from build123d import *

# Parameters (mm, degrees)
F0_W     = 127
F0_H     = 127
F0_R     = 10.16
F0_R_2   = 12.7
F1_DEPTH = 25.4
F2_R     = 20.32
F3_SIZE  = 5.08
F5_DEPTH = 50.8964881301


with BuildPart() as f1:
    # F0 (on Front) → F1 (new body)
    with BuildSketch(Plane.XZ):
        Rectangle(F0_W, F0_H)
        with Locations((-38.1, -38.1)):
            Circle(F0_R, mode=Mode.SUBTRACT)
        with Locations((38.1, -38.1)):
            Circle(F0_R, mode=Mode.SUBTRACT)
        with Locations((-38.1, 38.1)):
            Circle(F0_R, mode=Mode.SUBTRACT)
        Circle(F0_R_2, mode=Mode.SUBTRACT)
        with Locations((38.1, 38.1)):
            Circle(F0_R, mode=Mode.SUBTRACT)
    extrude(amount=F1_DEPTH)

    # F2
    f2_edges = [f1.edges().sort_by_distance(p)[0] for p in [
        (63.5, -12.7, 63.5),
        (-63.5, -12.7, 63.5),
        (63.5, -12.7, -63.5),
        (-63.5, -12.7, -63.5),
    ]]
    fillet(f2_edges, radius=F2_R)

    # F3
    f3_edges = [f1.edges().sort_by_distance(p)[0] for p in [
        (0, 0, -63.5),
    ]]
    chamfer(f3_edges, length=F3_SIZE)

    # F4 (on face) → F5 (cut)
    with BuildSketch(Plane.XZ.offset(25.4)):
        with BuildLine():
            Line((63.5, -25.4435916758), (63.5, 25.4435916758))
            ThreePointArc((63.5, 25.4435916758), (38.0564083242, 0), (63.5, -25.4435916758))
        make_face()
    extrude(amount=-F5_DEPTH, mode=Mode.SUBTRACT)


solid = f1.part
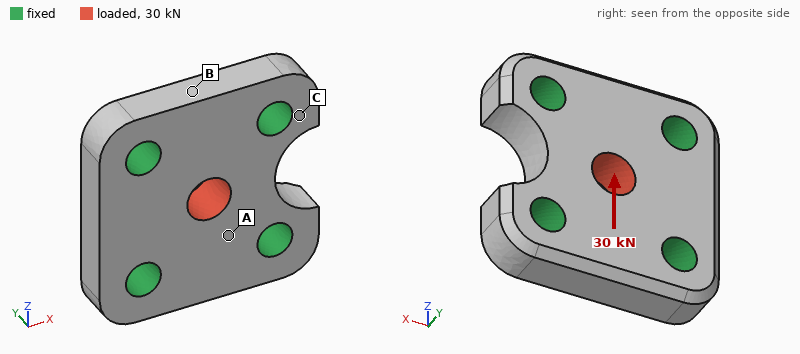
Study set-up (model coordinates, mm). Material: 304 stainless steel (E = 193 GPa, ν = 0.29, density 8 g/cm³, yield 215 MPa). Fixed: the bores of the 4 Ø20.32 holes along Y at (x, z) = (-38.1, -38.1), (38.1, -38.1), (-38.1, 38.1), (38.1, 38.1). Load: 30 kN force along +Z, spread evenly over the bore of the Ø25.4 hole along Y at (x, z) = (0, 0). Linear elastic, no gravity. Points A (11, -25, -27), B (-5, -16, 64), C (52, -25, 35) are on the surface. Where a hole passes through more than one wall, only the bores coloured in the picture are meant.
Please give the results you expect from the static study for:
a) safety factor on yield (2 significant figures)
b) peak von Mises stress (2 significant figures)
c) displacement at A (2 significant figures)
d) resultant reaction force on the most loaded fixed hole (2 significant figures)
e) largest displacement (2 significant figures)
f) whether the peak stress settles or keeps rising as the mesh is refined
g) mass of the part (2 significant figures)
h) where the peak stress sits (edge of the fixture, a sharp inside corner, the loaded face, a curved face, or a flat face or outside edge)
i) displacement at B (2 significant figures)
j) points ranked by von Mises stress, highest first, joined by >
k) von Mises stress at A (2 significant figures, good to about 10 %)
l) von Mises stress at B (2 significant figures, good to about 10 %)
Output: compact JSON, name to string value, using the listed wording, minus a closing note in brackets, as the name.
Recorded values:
{"safety factor on yield": "8.3", "peak von Mises stress": "26 MPa", "displacement at A": "1.6 µm", "resultant reaction force on the most loaded fixed hole": "8.2 kN", "largest displacement": "2.8 µm", "whether the peak stress settles or keeps rising as the mesh is refined": "settles", "mass of the part": "2.6 kg", "where the peak stress sits": "the loaded face", "displacement at B": "1.2 µm", "points ranked by von Mises stress, highest first, joined by >": "A > B > C", "von Mises stress at A": "9.5 MPa", "von Mises stress at B": "5.9 MPa"}
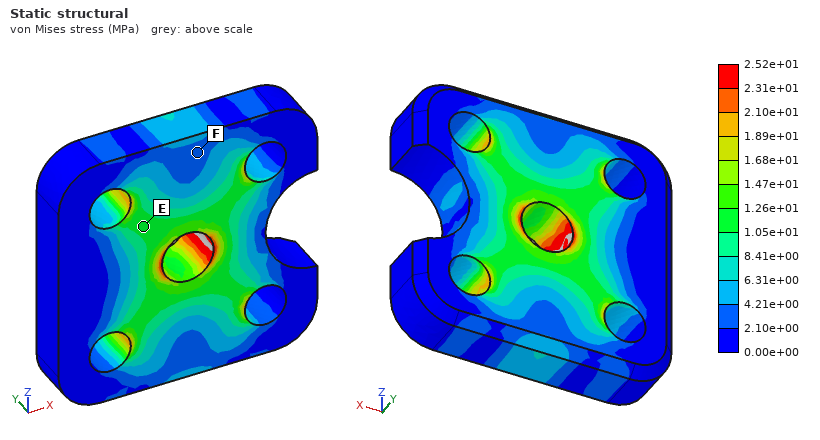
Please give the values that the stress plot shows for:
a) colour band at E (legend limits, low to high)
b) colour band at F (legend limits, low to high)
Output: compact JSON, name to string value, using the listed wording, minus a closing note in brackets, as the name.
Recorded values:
{"colour band at E": "1.05e+01 to 1.26e+01 MPa", "colour band at F": "2.10e+00 to 4.21e+00 MPa"}
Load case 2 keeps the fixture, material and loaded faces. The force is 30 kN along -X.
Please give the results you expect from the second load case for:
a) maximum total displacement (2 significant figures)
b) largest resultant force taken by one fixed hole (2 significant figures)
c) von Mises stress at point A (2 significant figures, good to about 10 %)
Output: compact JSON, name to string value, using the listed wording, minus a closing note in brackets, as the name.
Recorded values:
{"maximum total displacement": "3.1 µm", "largest resultant force taken by one fixed hole": "8.6 kN", "von Mises stress at point A": "8.3 MPa"}
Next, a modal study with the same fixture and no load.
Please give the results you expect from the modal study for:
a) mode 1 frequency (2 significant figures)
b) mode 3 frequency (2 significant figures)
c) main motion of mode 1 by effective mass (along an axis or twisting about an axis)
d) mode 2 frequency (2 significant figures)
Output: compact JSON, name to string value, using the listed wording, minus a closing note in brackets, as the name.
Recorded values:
{"mode 1 frequency": "15 kHz", "mode 3 frequency": "17 kHz", "main motion of mode 1 by effective mass": "along Y", "mode 2 frequency": "17 kHz"}
